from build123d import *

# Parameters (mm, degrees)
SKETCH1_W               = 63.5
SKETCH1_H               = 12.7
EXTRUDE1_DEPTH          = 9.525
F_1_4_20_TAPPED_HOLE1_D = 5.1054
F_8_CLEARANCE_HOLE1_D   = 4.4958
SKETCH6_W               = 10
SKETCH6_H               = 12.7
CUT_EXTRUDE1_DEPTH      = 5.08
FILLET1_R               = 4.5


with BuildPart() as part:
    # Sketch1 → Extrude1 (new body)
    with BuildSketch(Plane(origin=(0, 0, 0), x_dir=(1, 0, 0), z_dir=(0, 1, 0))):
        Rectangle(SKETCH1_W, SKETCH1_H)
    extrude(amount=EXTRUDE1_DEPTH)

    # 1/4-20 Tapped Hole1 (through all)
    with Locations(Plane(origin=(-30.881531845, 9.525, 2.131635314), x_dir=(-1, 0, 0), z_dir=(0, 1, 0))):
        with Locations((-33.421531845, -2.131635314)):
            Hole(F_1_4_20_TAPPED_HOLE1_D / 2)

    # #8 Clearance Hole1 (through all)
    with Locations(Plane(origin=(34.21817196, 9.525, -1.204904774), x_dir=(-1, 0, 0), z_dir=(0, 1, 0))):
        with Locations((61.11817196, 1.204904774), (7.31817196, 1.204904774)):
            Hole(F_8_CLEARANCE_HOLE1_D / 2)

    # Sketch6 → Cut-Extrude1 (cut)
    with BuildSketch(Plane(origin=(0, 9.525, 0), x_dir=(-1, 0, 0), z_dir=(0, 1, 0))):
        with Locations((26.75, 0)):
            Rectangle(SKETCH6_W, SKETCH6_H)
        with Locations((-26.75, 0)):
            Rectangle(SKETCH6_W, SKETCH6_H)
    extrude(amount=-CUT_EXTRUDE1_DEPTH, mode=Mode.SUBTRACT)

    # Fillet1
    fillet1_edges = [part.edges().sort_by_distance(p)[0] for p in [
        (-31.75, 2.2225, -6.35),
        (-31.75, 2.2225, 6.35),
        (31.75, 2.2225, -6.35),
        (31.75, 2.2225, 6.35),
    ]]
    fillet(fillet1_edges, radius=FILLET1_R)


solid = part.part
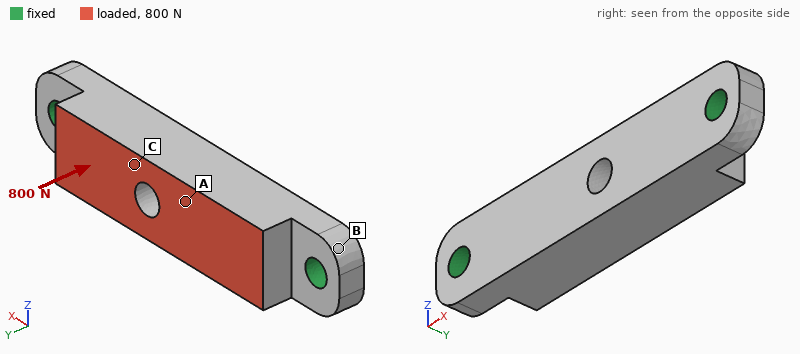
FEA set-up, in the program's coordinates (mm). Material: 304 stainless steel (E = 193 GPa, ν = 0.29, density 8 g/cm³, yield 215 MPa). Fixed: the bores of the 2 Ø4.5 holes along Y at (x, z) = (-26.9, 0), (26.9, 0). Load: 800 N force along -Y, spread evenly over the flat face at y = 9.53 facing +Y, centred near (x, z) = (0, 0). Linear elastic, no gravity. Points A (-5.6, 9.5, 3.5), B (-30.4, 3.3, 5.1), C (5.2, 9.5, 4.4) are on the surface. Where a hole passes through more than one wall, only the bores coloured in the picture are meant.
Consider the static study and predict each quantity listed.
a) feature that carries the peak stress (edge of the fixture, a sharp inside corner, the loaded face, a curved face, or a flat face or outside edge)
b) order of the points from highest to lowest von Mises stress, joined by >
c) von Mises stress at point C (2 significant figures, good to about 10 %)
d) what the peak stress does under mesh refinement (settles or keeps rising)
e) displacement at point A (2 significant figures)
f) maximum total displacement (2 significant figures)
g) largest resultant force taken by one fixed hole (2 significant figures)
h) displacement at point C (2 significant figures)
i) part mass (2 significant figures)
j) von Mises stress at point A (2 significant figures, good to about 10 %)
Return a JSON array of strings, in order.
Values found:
["edge of the fixture", "C > A > B", "26 MPa", "keeps rising", "5.1 µm", "5.7 µm", "570 N", "5.3 µm", "48 g", "17 MPa"]
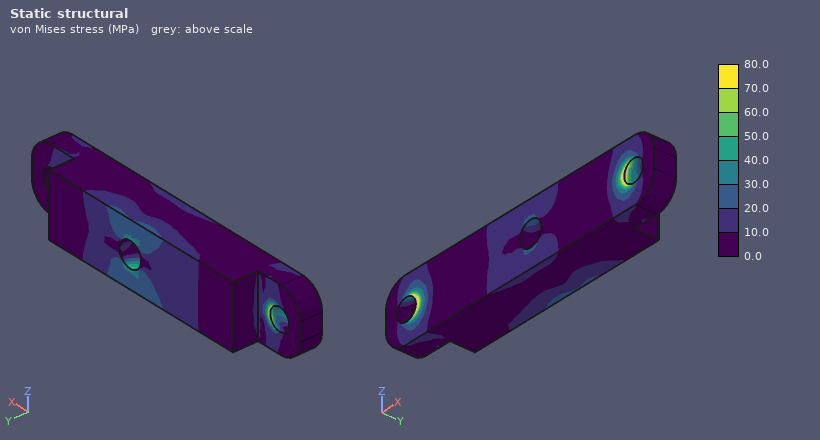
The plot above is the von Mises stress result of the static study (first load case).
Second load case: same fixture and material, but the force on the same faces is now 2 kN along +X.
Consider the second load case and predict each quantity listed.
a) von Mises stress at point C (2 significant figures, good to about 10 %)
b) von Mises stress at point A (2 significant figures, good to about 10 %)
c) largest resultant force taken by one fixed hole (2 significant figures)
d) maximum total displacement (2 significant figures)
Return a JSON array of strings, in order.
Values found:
["7.1 MPa", "6.7 MPa", "1.1 kN", "1.9 µm"]
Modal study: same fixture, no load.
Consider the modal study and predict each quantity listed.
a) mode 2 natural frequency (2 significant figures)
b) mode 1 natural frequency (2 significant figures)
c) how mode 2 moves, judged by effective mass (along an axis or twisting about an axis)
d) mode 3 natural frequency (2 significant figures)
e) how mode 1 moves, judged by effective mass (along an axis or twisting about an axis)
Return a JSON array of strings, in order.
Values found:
["11 kHz", "11 kHz", "along Z", "17 kHz", "along Y"]
